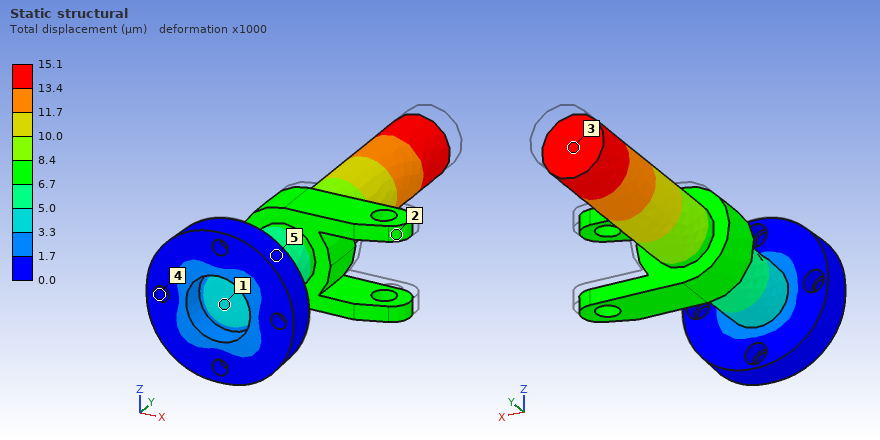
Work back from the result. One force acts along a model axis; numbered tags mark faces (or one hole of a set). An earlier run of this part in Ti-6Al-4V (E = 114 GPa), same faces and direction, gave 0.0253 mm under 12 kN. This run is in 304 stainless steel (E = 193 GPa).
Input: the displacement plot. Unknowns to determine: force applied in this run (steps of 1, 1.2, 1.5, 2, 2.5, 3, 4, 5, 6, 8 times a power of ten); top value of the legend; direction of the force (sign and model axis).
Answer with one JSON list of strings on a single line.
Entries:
["12 kN", "15.1 µm", "-Y"]
